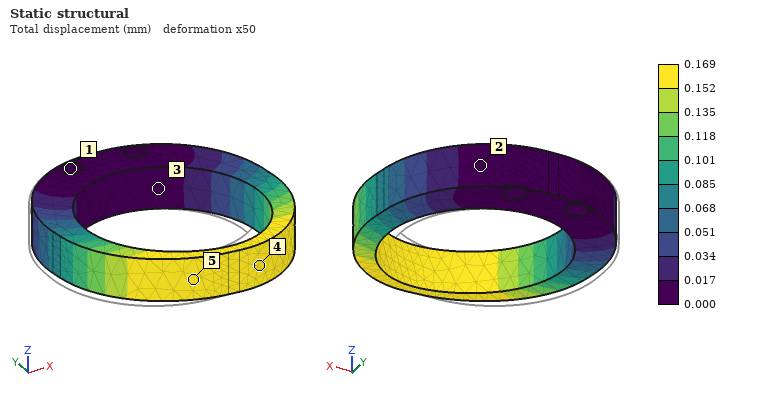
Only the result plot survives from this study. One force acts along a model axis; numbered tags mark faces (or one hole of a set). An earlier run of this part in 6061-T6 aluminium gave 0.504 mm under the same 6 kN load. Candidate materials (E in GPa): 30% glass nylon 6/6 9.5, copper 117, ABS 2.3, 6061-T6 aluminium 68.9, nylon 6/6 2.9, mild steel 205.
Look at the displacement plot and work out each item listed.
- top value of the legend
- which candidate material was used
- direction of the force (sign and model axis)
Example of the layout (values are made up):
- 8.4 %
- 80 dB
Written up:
- 0.169 mm
- mild steel
- +X
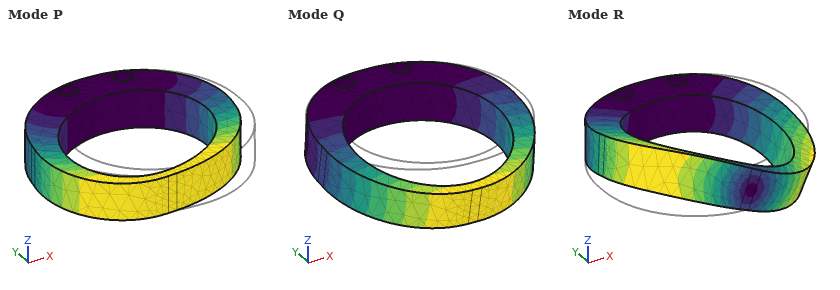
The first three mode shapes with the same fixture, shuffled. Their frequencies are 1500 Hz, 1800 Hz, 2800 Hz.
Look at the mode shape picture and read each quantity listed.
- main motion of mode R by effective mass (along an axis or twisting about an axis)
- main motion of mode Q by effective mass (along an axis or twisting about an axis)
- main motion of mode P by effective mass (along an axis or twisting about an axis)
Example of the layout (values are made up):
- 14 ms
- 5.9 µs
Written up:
- twisting about Y
- along Z
- along X
